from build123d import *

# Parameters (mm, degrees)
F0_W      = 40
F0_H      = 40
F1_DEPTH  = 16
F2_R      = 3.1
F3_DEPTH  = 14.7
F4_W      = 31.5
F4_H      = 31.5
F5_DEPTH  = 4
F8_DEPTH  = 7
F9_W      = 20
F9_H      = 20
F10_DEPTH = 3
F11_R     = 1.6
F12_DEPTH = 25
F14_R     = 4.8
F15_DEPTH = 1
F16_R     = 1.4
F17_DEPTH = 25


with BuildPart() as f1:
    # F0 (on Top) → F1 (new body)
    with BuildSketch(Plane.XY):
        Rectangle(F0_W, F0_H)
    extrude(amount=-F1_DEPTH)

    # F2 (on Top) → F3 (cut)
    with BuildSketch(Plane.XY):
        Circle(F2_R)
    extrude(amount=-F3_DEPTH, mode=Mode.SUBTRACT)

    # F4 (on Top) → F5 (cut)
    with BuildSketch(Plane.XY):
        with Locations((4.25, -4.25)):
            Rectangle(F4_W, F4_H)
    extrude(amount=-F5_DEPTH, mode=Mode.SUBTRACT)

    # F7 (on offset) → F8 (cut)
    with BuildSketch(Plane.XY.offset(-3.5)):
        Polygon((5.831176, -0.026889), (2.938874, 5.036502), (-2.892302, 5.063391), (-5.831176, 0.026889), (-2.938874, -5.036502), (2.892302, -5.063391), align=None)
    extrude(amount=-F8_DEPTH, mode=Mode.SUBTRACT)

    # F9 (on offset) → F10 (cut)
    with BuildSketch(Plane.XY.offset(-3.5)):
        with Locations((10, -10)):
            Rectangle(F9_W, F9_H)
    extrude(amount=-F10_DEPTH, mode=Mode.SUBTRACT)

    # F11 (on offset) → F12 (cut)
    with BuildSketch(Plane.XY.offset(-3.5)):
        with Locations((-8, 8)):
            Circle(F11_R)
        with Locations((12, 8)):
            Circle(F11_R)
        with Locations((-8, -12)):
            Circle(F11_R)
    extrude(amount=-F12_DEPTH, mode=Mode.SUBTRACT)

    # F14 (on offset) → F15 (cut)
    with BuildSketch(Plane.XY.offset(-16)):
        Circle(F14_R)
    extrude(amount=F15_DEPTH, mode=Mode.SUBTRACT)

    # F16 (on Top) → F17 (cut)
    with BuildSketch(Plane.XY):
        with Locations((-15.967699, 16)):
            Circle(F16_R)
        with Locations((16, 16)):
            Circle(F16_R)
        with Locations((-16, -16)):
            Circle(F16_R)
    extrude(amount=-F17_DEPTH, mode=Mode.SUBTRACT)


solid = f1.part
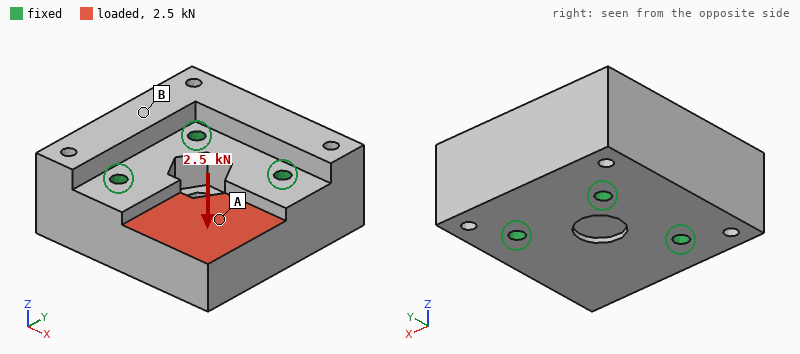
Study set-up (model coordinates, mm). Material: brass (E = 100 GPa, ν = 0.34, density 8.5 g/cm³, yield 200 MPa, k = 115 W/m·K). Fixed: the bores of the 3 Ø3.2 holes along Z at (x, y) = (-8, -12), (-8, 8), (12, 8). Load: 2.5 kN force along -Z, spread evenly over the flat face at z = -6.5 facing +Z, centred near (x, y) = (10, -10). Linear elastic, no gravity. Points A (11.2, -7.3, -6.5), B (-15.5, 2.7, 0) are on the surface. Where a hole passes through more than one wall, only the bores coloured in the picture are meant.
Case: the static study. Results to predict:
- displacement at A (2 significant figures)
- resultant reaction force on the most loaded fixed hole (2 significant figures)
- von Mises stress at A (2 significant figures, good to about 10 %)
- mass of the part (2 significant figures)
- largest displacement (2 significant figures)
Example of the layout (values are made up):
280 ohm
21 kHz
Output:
11 µm
1.4 kN
22 MPa
160 g
27 µm
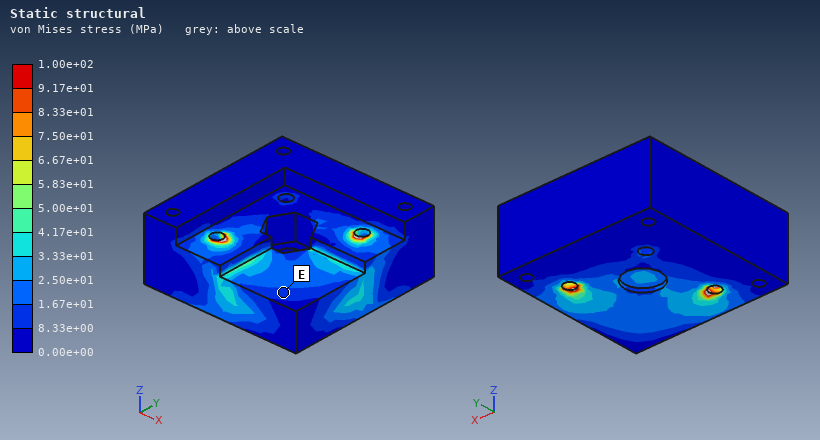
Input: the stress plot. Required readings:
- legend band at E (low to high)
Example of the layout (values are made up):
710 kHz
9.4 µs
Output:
8.33e+00 to 1.67e+01 MPa
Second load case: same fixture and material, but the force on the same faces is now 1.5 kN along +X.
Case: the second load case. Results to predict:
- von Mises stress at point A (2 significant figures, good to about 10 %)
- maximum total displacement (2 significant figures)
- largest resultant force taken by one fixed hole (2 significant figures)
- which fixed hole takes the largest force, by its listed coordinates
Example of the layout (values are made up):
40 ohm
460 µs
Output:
11 MPa
6.7 µm
1.1 kN
(-8, -12)
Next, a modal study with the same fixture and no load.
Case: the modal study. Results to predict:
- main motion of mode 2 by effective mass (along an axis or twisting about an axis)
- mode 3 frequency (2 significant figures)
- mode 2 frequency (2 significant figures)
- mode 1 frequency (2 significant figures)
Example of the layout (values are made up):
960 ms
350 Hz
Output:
along Z
20 kHz
20 kHz
12 kHz
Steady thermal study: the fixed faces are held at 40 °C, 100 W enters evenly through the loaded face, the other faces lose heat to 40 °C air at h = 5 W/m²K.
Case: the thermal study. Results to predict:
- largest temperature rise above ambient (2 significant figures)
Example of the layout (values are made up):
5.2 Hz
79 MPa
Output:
56 K
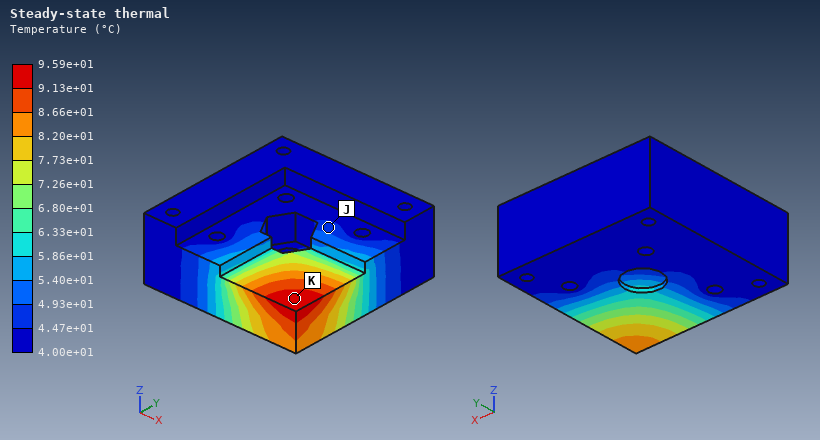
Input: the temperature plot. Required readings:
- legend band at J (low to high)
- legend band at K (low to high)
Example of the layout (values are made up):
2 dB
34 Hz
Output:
4.47e+01 to 4.93e+01 °C
9.13e+01 to 9.59e+01 °C
